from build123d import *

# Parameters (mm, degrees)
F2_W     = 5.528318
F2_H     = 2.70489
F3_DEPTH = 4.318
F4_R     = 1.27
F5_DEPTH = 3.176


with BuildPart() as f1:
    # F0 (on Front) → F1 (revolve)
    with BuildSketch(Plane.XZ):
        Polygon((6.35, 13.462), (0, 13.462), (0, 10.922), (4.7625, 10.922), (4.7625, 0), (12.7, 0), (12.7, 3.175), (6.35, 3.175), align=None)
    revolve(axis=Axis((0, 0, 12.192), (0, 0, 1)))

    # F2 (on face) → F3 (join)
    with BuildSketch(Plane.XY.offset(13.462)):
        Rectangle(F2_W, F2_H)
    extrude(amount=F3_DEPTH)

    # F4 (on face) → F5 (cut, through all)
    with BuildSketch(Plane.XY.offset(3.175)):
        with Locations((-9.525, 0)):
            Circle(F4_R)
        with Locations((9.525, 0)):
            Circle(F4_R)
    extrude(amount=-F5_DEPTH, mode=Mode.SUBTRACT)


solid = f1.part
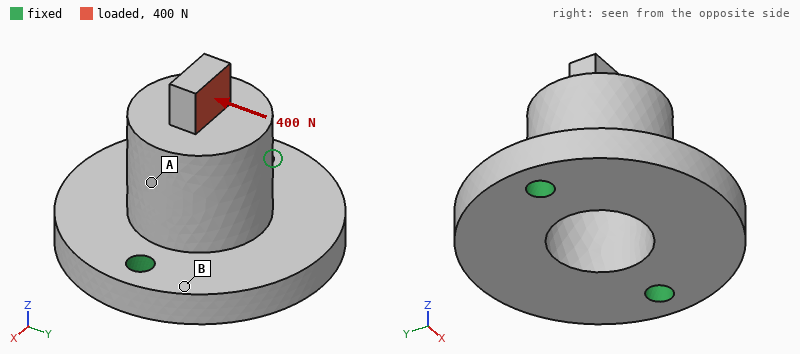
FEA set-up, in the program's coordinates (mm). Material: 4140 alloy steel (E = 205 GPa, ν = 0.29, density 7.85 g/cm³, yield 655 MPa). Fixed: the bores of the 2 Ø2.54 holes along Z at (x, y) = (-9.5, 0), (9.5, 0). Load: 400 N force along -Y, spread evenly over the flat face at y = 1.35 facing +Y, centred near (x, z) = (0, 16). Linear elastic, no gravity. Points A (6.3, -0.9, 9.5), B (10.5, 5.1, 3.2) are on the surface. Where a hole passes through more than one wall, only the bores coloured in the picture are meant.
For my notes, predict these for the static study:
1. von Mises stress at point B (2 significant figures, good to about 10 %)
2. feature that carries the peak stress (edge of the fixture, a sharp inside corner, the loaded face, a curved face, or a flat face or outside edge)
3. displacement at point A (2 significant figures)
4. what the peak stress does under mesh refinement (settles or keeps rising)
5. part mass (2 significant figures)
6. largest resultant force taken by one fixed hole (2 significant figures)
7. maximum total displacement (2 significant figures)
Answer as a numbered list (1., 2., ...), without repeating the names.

1. 44 MPa
2. edge of the fixture
3. 12 µm
4. keeps rising
5. 17 g
6. 200 N
7. 31 µm
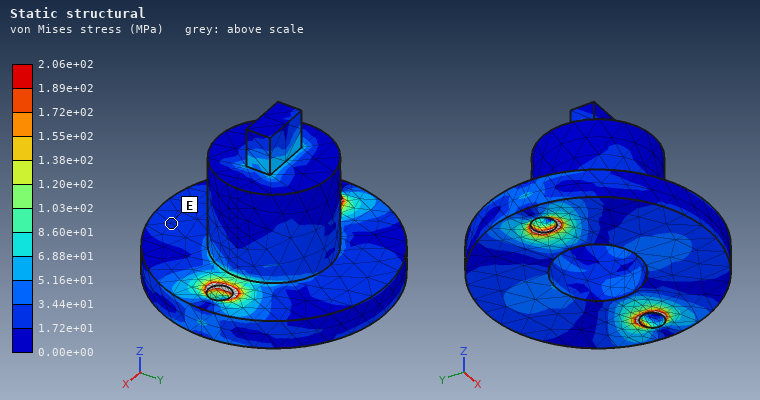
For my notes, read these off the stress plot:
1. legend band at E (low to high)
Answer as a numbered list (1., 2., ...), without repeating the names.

1. 1.72e+01 to 3.44e+01 MPa
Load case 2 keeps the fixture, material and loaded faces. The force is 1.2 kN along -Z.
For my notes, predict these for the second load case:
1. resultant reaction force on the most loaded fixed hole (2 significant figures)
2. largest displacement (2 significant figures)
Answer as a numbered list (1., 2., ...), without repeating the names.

1. 610 N
2. 20 µm
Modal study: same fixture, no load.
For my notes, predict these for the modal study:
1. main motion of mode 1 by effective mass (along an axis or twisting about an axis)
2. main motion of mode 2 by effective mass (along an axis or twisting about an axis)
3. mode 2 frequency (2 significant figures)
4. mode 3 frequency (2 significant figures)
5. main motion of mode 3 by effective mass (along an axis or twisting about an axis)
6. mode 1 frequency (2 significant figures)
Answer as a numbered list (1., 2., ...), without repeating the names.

1. along Y
2. along Z
3. 22 kHz
4. 24 kHz
5. along X
6. 10 kHz
